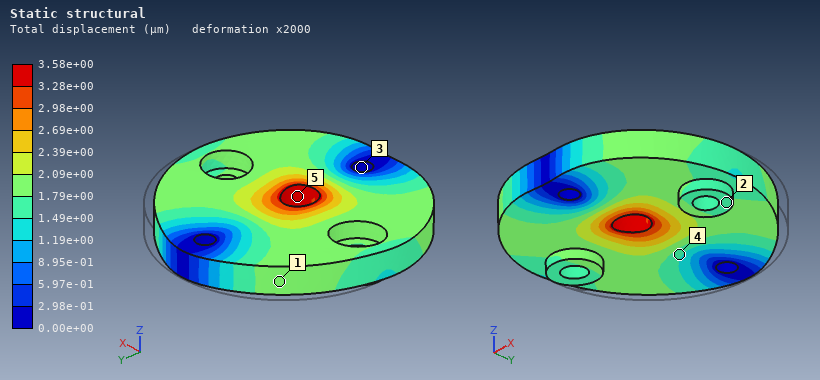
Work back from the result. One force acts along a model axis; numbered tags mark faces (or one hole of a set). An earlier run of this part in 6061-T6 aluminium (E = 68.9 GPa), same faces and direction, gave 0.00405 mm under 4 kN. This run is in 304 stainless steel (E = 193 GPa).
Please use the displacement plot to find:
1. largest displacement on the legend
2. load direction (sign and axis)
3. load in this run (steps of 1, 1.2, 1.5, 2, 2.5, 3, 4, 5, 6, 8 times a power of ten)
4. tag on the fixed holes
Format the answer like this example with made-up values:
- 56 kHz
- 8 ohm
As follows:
- 3.58e+00 µm
- -Y
- 10 kN
- 3
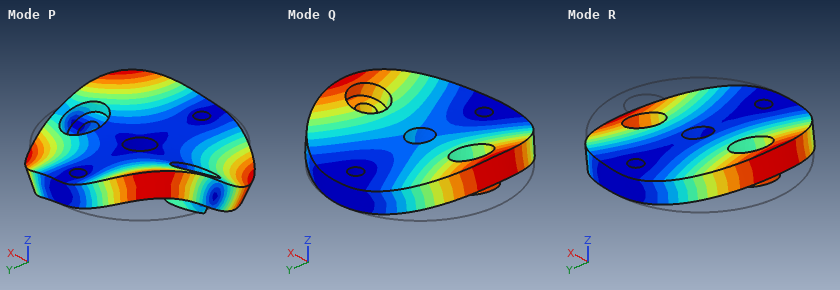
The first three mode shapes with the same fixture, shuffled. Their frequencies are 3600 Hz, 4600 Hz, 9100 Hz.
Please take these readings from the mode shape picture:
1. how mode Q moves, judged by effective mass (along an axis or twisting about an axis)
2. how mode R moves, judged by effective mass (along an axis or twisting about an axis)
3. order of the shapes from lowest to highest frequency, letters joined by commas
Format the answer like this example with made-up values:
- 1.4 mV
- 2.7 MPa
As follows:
- along Z
- twisting about Y
- R, Q, P
